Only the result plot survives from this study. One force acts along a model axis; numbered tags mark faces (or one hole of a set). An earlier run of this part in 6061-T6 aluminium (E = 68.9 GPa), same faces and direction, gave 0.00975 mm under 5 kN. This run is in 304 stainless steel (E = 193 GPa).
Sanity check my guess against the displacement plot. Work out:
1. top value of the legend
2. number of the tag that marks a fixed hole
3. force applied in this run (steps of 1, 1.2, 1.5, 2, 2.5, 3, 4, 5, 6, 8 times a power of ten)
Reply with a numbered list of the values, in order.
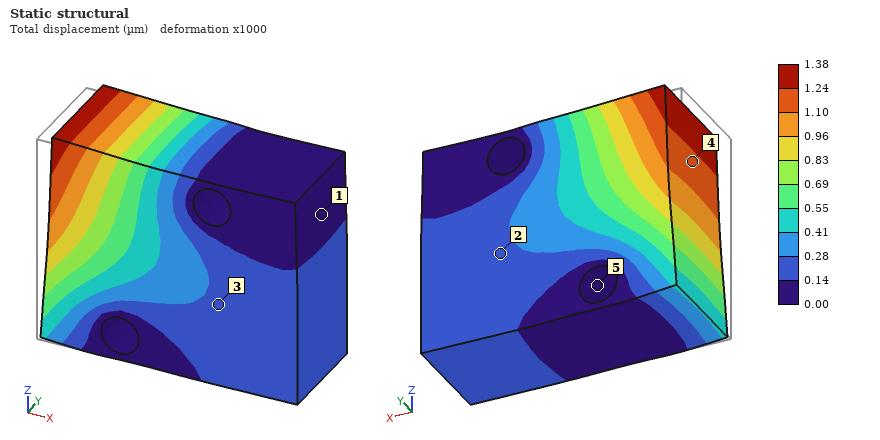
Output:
1. 1.38 µm
2. 5
3. 2 kN
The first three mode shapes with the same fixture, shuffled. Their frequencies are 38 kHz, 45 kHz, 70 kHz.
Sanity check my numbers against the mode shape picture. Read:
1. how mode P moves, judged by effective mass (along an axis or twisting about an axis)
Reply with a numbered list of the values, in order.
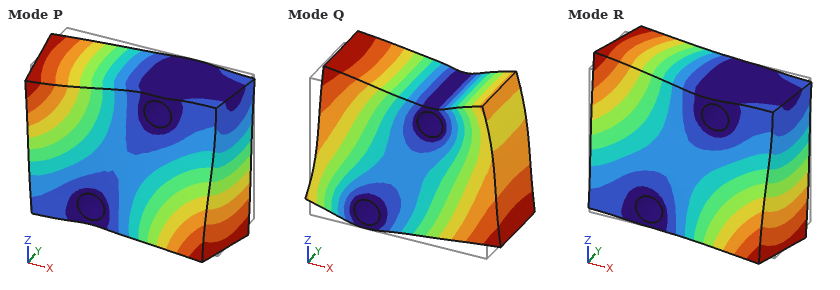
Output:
1. along Y
